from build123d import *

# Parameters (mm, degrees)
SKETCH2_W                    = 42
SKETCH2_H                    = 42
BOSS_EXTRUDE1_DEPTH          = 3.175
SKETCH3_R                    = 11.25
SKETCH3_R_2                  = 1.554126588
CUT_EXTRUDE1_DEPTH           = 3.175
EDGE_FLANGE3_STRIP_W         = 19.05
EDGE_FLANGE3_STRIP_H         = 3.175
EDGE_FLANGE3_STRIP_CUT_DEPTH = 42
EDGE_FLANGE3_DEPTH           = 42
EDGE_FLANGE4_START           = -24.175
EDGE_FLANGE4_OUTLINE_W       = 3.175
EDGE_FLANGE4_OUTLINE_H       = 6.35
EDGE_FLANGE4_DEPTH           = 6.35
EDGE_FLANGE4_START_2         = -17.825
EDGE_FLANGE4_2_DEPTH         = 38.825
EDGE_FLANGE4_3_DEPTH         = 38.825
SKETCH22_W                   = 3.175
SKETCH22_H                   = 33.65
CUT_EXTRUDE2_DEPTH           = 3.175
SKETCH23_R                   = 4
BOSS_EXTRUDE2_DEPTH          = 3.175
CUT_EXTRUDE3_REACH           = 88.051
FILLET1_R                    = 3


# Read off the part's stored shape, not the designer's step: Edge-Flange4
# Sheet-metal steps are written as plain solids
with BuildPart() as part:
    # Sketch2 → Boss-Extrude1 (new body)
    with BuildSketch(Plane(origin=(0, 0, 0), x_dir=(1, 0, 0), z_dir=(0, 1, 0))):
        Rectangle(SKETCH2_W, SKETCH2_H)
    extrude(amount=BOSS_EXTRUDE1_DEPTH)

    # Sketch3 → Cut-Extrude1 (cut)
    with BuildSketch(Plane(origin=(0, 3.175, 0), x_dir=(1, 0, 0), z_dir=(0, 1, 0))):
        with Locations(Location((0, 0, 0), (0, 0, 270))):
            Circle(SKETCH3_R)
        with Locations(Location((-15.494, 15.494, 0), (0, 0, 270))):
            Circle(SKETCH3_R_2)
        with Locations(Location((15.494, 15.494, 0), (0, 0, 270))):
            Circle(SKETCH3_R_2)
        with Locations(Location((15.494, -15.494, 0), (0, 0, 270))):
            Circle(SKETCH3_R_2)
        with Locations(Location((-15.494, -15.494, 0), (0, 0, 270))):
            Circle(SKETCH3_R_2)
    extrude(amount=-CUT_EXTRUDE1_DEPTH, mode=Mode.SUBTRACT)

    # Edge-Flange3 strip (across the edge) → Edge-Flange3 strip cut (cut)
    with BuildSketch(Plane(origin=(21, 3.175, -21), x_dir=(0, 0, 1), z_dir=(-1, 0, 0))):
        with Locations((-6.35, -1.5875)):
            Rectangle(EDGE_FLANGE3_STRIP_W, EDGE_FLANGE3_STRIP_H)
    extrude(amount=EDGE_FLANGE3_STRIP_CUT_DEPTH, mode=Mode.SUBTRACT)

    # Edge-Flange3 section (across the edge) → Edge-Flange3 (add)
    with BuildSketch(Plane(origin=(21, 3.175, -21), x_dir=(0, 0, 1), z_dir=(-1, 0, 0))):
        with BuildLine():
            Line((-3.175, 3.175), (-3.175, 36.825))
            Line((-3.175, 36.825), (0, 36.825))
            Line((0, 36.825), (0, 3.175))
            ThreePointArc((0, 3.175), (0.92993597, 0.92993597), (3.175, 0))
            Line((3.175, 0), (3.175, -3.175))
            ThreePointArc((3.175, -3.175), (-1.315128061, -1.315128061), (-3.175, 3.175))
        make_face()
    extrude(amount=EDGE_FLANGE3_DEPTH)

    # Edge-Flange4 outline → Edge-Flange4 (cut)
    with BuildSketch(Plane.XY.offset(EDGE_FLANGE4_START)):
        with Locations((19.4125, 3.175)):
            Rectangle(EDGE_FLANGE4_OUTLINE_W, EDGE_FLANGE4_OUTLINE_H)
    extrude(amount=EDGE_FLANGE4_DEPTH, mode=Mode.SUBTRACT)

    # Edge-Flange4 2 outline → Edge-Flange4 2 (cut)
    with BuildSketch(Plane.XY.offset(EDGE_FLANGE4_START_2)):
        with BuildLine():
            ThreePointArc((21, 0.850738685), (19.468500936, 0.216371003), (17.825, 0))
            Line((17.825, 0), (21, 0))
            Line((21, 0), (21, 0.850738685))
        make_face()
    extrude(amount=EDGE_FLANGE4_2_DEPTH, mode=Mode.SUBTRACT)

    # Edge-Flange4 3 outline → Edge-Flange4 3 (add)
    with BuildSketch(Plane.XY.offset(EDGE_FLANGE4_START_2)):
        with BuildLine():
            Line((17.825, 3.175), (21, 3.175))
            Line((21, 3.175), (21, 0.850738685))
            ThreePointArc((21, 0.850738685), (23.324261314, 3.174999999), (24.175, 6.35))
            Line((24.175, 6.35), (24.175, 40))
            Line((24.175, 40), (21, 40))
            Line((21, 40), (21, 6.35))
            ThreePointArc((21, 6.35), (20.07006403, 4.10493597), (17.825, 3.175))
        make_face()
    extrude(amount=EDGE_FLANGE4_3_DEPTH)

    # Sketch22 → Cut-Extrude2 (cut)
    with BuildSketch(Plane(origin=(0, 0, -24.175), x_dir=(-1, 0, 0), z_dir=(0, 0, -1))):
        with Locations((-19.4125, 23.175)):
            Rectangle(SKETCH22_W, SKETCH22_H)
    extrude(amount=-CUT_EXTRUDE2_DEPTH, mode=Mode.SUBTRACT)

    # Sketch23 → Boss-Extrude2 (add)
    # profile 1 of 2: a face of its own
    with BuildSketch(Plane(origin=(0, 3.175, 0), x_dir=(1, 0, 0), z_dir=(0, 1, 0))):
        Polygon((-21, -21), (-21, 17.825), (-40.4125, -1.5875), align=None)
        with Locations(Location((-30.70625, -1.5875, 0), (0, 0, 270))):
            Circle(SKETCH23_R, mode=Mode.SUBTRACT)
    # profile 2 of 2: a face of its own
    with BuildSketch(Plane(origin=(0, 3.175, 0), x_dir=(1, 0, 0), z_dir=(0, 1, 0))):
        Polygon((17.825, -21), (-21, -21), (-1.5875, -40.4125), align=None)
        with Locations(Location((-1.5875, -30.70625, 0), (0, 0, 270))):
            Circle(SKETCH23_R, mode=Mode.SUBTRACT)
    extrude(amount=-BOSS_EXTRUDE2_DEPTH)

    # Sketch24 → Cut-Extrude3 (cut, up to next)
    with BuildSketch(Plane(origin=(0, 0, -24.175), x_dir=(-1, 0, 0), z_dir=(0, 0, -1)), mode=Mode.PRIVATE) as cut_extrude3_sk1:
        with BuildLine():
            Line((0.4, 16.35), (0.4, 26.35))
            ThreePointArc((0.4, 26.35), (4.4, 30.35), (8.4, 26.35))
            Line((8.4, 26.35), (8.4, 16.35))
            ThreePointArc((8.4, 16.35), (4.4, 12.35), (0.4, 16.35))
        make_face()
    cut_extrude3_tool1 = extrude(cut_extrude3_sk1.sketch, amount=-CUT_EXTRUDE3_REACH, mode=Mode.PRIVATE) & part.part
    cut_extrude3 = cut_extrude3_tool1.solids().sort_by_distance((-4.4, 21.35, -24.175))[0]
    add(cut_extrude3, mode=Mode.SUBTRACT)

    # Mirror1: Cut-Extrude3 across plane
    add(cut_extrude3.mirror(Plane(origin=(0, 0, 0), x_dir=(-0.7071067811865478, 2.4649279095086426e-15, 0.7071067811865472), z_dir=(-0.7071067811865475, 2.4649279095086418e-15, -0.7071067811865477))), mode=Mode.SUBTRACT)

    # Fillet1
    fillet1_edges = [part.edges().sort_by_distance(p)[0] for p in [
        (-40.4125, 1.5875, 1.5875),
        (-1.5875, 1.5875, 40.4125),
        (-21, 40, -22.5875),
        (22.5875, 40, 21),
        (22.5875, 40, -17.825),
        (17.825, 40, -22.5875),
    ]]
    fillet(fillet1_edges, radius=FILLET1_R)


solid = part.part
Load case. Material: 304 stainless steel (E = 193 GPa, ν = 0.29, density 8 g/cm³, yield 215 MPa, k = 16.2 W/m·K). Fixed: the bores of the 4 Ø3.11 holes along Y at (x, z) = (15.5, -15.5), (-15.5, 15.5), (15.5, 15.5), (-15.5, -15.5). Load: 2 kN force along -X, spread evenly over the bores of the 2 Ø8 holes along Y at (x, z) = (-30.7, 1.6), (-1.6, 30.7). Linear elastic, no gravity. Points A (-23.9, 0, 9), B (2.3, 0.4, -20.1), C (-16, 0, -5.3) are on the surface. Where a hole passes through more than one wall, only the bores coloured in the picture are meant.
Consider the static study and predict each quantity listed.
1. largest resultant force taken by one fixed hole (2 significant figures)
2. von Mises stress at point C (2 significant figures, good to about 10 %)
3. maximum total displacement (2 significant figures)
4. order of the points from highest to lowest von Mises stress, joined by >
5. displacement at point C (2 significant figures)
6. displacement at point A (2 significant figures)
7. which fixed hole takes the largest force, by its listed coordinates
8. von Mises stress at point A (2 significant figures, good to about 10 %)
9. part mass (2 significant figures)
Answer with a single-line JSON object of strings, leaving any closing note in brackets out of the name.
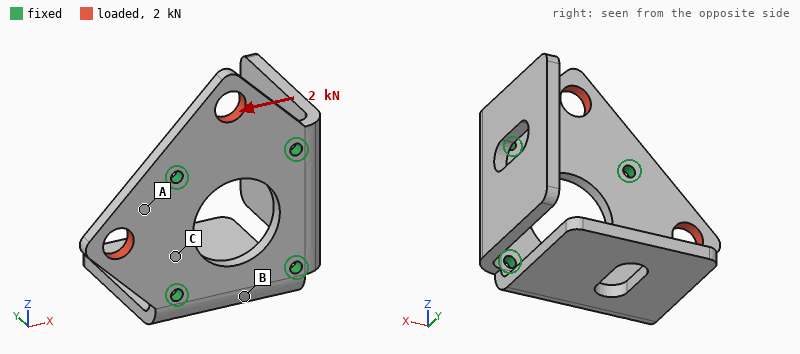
{"largest resultant force taken by one fixed hole": "1.2 kN", "von Mises stress at point C": "10 MPa", "maximum total displacement": "5.5 µm", "order of the points from highest to lowest von Mises stress, joined by >": "A > C > B", "displacement at point C": "1.2 µm", "displacement at point A": "1.3 µm", "which fixed hole takes the largest force, by its listed coordinates": "(-15.5, 15.5)", "von Mises stress at point A": "18 MPa", "part mass": "120 g"}
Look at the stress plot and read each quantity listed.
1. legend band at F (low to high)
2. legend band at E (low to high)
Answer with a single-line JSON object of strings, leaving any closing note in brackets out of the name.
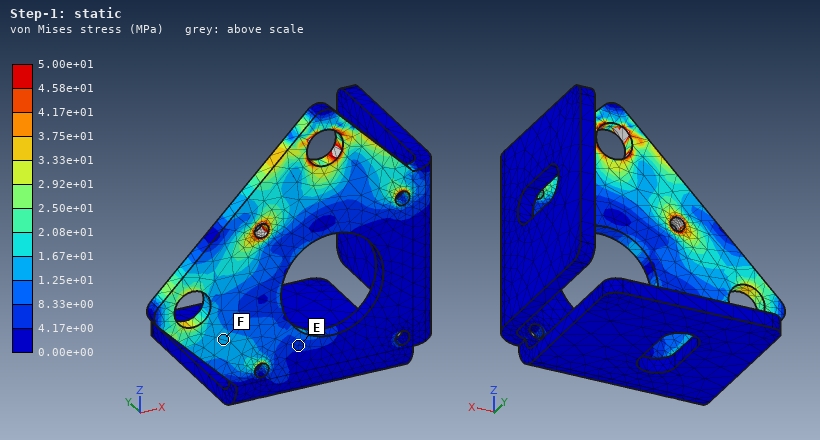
{"legend band at F": "1.25e+01 to 1.67e+01 MPa", "legend band at E": "4.17e+00 to 8.33e+00 MPa"}
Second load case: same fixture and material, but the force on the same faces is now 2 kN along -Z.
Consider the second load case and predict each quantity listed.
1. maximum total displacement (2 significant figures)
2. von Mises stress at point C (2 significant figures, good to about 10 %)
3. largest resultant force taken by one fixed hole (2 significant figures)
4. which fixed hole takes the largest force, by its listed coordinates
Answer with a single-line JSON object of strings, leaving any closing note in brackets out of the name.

{"maximum total displacement": "5.5 µm", "von Mises stress at point C": "7.3 MPa", "largest resultant force taken by one fixed hole": "1.2 kN", "which fixed hole takes the largest force, by its listed coordinates": "(-15.5, 15.5)"}
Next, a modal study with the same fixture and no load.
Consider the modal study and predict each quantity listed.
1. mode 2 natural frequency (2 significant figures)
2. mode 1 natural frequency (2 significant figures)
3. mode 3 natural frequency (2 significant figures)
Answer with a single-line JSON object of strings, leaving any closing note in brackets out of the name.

{"mode 2 natural frequency": "1400 Hz", "mode 1 natural frequency": "1300 Hz", "mode 3 natural frequency": "3500 Hz"}
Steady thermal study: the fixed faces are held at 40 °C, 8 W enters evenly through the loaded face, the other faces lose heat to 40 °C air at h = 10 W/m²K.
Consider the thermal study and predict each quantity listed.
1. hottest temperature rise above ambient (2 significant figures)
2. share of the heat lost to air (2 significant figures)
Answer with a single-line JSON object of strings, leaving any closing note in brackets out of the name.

{"hottest temperature rise above ambient": "78 K", "share of the heat lost to air": "12 %"}
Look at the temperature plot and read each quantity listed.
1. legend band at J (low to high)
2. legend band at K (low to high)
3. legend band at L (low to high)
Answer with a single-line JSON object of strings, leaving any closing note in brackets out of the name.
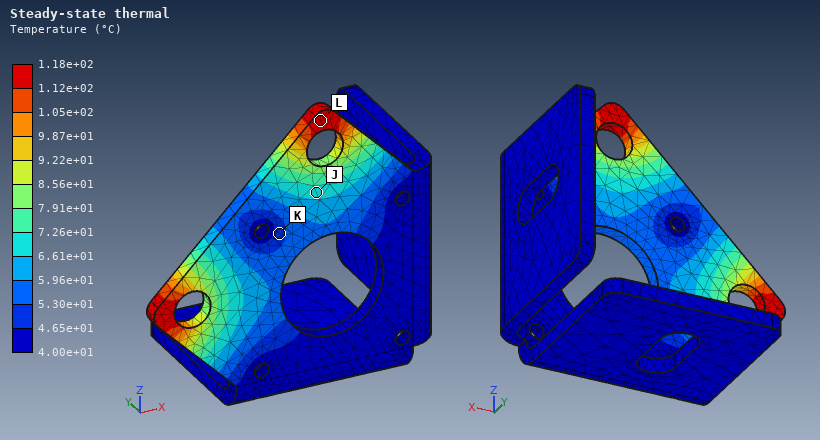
{"legend band at J": "6.61e+01 to 7.26e+01 °C", "legend band at K": "4.65e+01 to 5.30e+01 °C", "legend band at L": "1.12e+02 to 1.18e+02 °C"}
